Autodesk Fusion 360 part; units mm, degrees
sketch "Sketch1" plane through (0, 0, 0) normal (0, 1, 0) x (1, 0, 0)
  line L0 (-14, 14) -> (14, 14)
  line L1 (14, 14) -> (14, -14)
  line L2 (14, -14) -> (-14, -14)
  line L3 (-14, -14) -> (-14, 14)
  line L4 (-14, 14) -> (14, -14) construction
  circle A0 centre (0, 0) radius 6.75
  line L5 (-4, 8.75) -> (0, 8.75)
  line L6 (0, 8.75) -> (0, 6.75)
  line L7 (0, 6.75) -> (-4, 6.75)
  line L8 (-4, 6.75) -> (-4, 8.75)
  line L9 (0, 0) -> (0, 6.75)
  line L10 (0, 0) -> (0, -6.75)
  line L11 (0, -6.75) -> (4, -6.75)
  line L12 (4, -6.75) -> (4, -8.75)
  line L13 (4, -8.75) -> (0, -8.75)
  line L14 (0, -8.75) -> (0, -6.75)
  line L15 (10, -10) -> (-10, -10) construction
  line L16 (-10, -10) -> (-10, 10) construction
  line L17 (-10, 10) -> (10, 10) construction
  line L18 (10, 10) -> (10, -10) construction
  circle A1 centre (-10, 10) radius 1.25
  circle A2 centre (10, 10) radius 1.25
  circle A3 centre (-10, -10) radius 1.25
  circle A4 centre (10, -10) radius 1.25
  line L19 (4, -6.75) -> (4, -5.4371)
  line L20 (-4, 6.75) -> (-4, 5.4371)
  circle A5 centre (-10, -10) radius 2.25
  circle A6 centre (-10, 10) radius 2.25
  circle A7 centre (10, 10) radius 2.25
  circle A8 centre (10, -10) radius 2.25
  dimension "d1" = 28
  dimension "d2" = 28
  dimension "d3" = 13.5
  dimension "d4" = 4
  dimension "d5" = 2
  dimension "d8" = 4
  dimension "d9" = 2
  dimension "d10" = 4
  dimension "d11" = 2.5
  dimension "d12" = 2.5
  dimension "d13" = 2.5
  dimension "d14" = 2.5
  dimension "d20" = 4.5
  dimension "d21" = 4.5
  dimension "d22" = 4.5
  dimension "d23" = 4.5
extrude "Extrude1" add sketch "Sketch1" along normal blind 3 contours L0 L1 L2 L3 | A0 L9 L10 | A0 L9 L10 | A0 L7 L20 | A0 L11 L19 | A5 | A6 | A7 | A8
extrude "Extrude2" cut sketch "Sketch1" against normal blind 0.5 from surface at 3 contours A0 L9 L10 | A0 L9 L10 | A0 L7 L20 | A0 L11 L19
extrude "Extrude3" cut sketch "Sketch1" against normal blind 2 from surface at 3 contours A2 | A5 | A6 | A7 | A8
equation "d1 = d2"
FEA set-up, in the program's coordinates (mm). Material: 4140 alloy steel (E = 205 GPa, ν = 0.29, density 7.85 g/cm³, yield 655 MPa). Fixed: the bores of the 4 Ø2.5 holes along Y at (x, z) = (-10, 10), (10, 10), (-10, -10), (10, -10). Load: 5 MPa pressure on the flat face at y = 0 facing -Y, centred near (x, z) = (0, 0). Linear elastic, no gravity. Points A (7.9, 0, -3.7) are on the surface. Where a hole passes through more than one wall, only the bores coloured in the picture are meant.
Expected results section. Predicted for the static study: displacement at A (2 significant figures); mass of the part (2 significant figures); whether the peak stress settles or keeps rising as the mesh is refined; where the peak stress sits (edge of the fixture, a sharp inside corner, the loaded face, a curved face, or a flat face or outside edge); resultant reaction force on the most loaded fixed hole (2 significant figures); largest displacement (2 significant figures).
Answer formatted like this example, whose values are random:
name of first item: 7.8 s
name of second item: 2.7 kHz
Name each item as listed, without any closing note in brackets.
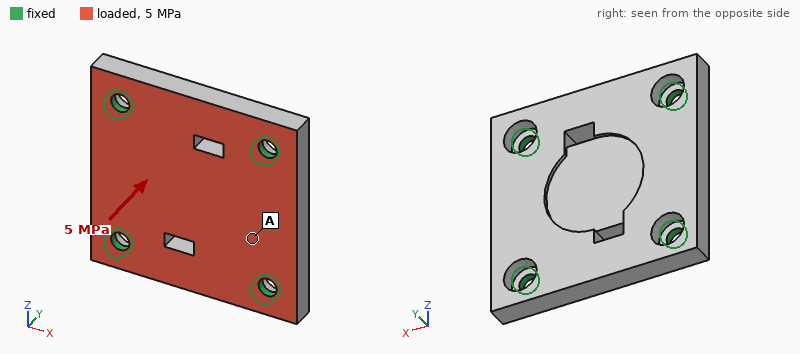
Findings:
displacement at A: 13 µm
mass of the part: 16 g
whether the peak stress settles or keeps rising as the mesh is refined: keeps rising
where the peak stress sits: edge of the fixture
resultant reaction force on the most loaded fixed hole: 1.1 kN
largest displacement: 23 µm
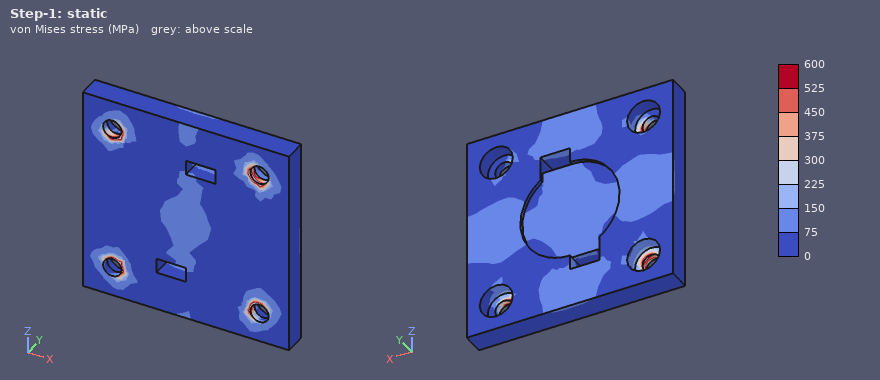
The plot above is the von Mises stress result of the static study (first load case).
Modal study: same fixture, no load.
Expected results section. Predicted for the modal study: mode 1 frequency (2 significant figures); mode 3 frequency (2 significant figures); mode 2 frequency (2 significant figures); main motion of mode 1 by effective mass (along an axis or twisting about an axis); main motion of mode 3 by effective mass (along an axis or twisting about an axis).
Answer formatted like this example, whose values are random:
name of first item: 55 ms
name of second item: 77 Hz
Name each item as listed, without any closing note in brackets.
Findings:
mode 1 frequency: 19 kHz
mode 3 frequency: 28 kHz
mode 2 frequency: 27 kHz
main motion of mode 1 by effective mass: along Y
main motion of mode 3 by effective mass: twisting about Z
